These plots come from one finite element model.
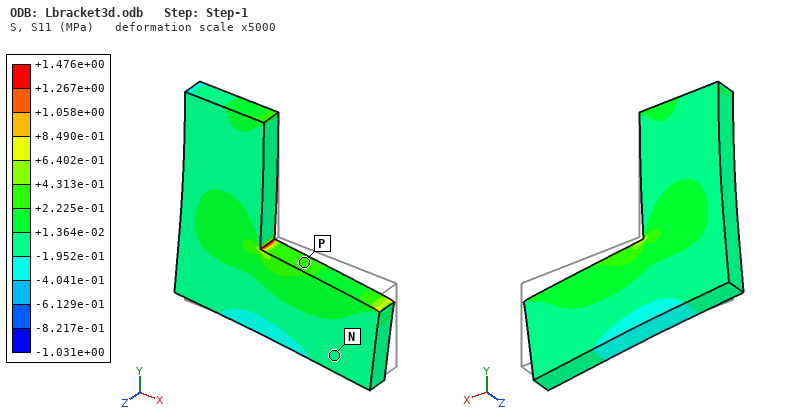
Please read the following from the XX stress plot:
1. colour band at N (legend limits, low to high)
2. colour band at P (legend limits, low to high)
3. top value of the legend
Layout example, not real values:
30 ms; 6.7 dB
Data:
-1.952e-01 to +1.364e-02 MPa; +2.225e-01 to +4.313e-01 MPa; +1.476e+00 MPa
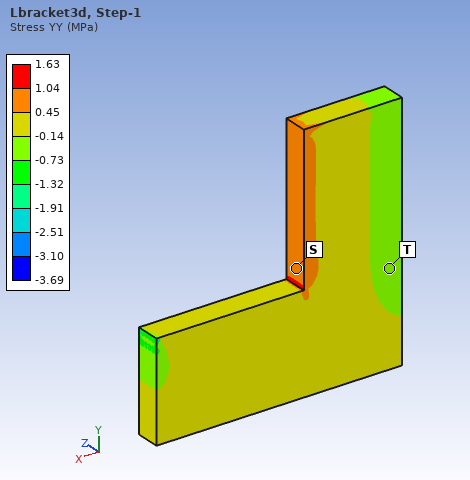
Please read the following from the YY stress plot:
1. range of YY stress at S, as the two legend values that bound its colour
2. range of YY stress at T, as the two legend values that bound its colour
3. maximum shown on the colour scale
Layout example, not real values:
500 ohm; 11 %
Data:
0.45 to 1.04 MPa; -0.73 to -0.14 MPa; 1.63 MPa
